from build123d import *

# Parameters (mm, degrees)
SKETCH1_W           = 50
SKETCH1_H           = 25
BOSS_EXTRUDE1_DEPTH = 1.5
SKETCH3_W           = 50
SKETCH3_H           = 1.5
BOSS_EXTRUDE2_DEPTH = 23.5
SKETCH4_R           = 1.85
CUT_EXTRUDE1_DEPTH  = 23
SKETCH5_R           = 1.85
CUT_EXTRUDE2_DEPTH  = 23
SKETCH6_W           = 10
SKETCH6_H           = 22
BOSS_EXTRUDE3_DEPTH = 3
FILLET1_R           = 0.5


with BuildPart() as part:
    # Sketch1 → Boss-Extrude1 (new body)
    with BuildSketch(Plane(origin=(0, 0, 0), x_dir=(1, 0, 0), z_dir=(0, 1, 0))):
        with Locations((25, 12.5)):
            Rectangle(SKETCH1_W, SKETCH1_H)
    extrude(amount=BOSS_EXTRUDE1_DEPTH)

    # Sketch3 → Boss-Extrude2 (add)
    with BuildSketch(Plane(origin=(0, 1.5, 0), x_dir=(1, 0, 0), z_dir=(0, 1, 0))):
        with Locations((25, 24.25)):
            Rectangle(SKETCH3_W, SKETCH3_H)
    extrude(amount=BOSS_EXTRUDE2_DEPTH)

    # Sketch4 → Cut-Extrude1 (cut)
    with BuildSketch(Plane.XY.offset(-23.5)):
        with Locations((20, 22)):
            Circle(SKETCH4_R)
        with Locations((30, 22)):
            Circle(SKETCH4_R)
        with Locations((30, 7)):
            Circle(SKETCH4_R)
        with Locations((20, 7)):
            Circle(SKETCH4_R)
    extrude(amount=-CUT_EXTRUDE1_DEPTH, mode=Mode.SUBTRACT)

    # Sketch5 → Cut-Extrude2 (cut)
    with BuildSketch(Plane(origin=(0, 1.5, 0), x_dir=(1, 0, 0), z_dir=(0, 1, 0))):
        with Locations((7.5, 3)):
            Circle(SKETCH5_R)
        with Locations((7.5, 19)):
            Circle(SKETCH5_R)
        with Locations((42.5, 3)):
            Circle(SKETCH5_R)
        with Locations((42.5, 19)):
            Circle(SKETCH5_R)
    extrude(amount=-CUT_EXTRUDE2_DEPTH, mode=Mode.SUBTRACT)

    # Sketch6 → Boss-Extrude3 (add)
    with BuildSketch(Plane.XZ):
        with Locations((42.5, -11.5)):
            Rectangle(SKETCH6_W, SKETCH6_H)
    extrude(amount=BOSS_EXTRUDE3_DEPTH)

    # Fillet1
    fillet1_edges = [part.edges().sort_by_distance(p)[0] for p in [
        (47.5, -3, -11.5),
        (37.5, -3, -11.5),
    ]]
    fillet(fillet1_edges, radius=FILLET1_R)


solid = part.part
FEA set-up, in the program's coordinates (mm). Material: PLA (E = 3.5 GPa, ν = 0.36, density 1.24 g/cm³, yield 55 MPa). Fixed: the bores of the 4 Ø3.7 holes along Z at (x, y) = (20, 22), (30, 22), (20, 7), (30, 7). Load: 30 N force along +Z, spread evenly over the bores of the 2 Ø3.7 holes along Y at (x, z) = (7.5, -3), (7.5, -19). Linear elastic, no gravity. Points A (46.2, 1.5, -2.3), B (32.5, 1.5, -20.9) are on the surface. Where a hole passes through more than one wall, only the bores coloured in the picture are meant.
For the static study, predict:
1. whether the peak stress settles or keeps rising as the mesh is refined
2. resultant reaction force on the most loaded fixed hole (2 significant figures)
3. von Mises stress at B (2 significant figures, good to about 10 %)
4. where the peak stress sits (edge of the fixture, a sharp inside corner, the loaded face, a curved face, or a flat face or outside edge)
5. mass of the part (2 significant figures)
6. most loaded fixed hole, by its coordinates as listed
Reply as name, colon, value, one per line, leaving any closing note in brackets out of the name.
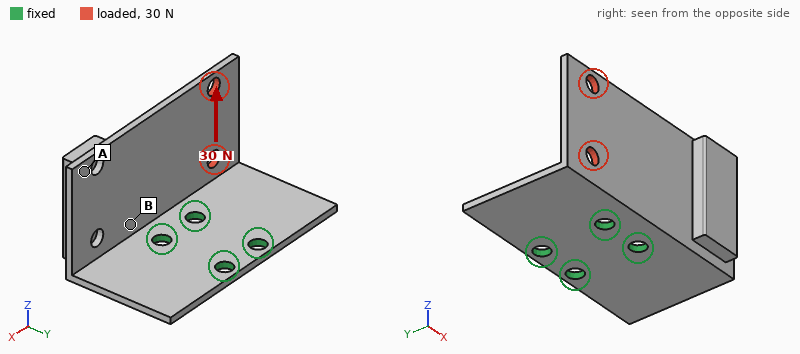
whether the peak stress settles or keeps rising as the mesh is refined: keeps rising
resultant reaction force on the most loaded fixed hole: 54 N
von Mises stress at B: 4.8 MPa
where the peak stress sits: edge of the fixture
mass of the part: 5.2 g
most loaded fixed hole, by its coordinates as listed: (20, 7)
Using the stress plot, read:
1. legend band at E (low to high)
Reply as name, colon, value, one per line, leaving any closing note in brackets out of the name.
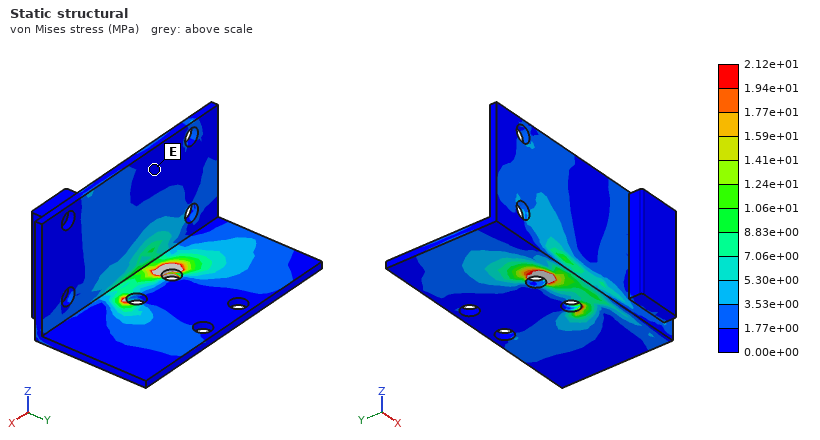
legend band at E: 0.00e+00 to 1.77e+00 MPa
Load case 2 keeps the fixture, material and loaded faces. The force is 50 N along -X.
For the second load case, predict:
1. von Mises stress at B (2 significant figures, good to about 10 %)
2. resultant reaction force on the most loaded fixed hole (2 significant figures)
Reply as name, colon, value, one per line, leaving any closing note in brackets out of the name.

von Mises stress at B: 7.5 MPa
resultant reaction force on the most loaded fixed hole: 57 N
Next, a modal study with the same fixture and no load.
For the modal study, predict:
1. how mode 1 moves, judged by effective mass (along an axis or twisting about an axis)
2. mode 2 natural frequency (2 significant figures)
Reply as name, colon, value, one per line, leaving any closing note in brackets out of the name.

how mode 1 moves, judged by effective mass: along Y
mode 2 natural frequency: 760 Hz
